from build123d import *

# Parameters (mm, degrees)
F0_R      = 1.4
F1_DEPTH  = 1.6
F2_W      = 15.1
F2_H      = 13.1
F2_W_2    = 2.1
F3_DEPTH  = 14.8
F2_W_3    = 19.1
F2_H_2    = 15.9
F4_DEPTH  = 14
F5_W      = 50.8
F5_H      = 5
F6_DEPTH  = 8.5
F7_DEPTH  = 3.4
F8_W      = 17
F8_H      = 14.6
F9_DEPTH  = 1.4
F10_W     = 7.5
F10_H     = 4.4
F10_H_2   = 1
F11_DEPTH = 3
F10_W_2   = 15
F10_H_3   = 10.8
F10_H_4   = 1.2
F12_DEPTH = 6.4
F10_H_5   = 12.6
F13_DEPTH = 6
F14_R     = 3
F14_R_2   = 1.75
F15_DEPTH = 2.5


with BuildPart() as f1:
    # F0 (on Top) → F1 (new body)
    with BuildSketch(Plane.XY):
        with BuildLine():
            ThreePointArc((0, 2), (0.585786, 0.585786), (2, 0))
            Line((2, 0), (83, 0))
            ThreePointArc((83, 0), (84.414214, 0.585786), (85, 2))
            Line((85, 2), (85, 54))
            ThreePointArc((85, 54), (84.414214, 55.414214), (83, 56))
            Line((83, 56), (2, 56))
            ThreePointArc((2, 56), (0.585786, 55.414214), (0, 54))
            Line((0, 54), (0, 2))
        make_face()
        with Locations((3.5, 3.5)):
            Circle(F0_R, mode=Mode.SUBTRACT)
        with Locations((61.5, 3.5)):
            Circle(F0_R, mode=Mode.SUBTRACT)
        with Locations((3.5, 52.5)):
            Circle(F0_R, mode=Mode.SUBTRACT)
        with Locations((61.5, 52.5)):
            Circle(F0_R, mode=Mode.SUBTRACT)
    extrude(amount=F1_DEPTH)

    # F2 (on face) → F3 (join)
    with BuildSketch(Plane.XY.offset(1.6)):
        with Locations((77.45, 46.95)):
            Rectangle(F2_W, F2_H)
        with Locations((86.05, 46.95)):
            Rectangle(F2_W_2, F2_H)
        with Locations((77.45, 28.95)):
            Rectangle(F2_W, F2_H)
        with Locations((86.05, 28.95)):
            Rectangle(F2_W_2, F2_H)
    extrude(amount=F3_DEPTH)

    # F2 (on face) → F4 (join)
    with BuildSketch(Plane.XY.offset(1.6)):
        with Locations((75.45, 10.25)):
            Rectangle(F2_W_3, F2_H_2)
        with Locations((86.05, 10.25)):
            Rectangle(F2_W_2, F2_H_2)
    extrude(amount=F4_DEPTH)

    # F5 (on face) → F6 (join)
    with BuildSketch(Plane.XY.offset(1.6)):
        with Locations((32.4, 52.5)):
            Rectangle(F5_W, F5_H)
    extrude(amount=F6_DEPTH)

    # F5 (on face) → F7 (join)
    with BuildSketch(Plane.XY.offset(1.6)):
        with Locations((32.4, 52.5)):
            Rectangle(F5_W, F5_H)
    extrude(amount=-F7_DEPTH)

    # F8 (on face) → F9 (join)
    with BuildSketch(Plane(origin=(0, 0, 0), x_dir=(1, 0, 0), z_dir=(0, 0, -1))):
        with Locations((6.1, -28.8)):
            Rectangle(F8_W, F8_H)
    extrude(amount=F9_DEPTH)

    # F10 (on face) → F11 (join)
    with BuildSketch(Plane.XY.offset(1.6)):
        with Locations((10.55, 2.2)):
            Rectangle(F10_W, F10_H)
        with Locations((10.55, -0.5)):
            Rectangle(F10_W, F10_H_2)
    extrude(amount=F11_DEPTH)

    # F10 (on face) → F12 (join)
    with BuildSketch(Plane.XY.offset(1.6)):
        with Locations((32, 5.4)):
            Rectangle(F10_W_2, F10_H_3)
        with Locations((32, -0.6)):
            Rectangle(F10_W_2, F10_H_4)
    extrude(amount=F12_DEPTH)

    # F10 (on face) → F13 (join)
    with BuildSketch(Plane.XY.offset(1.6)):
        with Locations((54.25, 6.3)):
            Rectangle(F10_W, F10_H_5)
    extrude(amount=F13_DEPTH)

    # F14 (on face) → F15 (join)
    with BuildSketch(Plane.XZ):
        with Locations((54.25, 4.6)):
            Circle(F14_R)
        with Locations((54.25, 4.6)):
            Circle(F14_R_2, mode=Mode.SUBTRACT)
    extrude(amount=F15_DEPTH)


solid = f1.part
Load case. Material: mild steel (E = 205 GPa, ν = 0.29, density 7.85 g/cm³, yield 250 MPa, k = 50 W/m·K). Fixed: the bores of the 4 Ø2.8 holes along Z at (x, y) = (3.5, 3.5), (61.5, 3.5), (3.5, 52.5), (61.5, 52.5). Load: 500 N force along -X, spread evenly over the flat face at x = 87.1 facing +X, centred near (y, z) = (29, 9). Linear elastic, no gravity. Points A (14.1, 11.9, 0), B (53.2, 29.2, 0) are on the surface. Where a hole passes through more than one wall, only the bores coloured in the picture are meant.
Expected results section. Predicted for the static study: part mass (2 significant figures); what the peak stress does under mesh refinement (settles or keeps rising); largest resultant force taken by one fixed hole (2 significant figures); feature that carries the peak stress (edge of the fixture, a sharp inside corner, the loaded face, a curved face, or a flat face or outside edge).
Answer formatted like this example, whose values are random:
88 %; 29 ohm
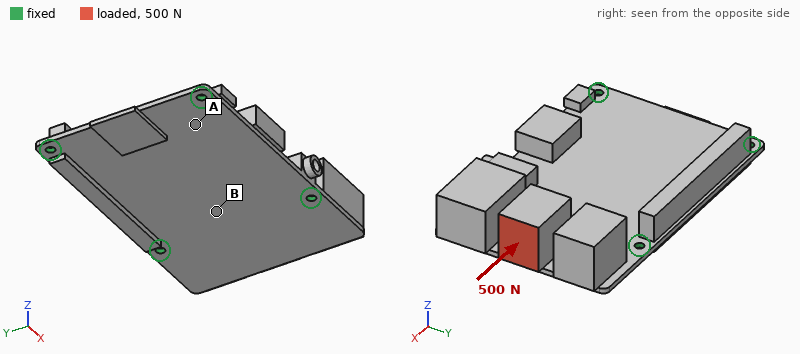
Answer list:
190 g; keeps rising; 180 N; edge of the fixture
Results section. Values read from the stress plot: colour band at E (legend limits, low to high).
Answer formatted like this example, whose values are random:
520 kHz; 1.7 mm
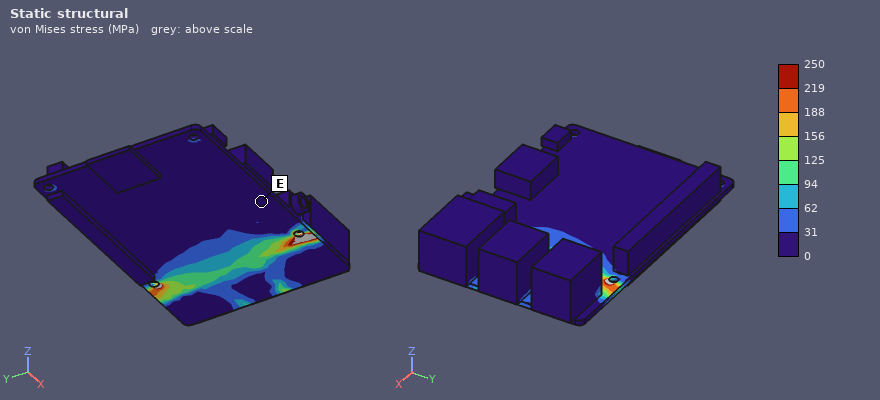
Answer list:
0 to 31 MPa
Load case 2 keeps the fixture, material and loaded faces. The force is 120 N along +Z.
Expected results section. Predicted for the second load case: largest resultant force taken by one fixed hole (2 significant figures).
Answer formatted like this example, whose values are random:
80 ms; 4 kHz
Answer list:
74 N
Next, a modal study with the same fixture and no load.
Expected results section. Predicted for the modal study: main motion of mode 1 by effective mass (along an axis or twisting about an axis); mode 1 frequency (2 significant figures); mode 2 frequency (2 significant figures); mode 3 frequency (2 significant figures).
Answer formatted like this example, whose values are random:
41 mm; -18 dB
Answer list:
along Z; 590 Hz; 1900 Hz; 2100 Hz
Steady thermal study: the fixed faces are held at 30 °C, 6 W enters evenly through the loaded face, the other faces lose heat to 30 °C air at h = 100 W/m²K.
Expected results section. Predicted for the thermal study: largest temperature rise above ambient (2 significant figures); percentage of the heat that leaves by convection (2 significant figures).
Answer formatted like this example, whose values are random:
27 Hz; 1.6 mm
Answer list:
21 K; 80 %
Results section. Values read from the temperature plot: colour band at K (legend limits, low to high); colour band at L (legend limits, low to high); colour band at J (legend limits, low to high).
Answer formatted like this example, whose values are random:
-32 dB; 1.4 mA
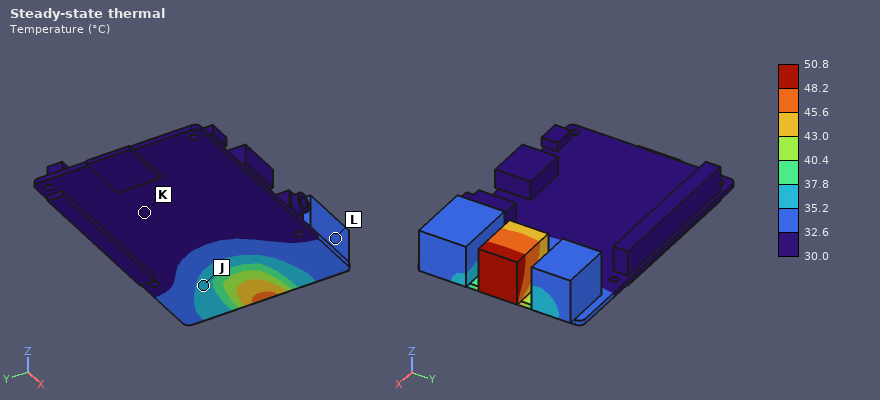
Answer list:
30.0 to 32.6 °C; 32.6 to 35.2 °C; 35.2 to 37.8 °C
